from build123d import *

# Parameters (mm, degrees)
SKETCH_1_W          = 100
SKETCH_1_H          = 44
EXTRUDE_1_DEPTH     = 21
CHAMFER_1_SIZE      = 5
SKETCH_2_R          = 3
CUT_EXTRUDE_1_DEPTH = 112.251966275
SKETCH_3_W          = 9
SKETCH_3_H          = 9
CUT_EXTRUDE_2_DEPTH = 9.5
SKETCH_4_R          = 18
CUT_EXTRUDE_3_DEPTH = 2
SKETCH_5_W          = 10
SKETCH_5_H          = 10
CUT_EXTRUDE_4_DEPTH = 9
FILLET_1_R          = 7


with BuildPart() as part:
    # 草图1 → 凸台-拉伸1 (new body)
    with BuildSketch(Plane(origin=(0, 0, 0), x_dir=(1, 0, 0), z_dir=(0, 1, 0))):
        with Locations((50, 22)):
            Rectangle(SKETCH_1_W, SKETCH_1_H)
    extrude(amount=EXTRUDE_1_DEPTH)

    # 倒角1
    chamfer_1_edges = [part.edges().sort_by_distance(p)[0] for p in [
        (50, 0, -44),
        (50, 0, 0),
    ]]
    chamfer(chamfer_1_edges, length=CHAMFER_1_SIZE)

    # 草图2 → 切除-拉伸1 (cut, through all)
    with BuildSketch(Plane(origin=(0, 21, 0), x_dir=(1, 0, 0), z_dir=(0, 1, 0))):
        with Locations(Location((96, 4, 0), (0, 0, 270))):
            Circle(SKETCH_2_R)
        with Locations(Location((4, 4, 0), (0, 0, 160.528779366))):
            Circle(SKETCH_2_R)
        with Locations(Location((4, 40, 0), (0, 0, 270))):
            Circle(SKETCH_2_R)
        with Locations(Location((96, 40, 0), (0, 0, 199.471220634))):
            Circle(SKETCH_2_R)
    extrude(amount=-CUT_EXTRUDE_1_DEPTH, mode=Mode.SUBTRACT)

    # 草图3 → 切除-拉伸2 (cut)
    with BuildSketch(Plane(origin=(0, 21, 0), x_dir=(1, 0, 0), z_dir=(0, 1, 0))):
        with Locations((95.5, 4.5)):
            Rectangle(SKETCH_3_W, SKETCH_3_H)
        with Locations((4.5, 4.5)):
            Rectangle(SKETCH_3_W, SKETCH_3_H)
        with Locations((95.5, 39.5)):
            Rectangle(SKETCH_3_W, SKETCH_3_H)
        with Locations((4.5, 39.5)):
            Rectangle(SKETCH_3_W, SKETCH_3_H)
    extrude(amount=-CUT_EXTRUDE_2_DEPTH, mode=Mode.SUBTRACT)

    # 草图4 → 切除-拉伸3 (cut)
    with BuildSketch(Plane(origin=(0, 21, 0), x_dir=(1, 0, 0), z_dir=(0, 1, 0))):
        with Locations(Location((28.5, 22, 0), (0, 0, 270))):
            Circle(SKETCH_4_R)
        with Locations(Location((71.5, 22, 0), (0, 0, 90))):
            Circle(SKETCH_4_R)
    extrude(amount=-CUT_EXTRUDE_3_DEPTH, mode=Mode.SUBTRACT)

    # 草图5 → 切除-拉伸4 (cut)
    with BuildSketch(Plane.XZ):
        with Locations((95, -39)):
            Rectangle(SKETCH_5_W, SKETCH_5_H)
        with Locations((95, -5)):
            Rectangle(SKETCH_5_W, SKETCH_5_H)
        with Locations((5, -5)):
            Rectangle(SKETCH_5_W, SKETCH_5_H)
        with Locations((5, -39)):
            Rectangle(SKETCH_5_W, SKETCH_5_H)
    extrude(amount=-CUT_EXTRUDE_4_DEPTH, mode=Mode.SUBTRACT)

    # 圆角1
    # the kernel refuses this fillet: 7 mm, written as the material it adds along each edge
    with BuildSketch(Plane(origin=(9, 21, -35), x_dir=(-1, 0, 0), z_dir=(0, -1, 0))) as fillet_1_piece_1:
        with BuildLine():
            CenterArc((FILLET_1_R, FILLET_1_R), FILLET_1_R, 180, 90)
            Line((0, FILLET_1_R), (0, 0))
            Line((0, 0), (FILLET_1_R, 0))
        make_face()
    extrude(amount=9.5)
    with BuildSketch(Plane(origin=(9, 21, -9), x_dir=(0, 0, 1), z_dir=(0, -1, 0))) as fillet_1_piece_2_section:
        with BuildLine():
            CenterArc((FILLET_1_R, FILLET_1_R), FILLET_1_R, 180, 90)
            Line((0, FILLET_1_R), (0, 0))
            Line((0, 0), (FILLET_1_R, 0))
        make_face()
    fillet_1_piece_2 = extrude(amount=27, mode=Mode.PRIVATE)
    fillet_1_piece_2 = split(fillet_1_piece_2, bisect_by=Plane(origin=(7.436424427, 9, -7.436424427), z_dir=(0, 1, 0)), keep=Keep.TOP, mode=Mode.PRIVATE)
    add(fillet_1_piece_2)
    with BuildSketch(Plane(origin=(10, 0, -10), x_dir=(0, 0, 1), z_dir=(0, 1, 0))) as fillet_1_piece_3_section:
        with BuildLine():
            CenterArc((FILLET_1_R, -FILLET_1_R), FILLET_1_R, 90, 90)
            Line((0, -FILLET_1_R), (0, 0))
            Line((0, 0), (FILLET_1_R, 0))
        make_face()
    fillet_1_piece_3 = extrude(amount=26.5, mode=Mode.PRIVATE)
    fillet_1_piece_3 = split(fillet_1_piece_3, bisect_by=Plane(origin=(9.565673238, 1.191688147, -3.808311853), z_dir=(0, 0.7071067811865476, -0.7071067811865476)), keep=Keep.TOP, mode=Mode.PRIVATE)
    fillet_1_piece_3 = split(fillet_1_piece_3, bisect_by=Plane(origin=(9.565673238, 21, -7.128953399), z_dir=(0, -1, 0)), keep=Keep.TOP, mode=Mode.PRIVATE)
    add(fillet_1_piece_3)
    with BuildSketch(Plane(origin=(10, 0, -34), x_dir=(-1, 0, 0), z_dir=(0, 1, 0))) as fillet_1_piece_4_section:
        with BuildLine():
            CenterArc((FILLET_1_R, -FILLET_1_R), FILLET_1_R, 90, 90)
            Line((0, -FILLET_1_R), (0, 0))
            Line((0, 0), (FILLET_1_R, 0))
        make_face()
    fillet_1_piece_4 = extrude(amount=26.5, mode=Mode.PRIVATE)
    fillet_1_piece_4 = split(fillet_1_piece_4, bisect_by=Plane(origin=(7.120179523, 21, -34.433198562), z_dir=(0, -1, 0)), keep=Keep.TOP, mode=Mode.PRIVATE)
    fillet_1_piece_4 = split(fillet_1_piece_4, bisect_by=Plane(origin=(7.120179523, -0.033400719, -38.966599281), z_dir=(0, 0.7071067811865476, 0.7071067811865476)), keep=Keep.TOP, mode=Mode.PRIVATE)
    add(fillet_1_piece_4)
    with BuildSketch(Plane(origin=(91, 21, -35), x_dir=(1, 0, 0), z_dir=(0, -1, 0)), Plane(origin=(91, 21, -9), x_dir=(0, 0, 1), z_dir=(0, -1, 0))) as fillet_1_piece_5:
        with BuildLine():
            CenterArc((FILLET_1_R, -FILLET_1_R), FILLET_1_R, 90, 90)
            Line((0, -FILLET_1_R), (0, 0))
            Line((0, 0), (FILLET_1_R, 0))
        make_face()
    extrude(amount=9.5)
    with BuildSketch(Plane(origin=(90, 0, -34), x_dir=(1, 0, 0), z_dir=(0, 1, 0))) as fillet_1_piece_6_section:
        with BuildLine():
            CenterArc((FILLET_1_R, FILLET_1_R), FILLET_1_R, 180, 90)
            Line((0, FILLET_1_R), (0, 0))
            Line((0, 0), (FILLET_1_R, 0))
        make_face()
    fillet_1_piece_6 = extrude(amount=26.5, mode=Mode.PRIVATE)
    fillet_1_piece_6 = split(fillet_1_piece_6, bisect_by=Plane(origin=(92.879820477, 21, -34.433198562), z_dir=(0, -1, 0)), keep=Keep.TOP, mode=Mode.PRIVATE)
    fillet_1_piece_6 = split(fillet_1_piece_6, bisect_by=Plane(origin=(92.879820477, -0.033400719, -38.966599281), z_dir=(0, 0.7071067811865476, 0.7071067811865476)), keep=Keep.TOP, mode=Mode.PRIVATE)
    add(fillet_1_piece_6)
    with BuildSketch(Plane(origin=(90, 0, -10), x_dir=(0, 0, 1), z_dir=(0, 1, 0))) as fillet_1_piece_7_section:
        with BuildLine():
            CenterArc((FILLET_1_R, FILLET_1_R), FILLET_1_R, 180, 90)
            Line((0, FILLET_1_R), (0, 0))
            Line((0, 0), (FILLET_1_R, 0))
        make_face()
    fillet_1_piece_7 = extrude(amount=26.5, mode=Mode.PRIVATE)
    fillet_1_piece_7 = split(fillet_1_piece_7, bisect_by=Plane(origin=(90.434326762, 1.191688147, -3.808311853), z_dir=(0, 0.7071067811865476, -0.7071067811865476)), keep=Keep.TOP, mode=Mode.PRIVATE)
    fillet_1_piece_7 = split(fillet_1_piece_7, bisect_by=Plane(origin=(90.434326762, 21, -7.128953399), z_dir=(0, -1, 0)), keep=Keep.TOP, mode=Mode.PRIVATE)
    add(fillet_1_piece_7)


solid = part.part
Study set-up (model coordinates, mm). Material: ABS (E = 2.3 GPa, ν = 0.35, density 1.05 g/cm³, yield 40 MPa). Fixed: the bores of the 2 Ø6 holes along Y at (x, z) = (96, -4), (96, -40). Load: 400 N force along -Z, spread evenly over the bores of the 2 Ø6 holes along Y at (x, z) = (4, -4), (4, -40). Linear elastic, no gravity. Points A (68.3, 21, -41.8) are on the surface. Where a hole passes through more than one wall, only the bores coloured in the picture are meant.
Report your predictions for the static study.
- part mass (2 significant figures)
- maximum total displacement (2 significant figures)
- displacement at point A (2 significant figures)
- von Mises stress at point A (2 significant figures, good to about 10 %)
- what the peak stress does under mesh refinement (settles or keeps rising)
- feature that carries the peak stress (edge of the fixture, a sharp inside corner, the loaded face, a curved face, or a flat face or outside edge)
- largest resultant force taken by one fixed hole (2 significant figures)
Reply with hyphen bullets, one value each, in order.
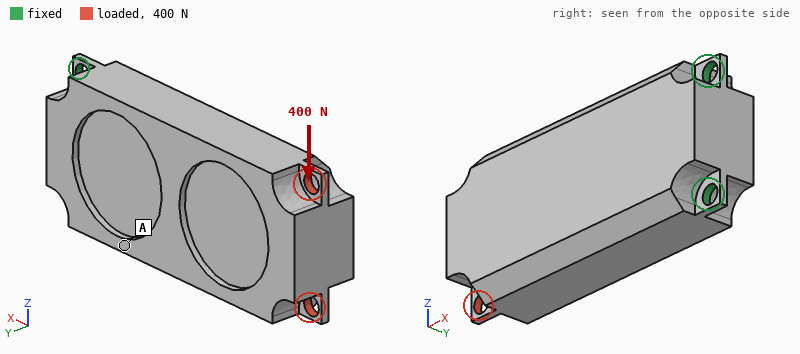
- 84 g
- 0.93 mm
- 0.21 mm
- 4.0 MPa
- keeps rising
- edge of the fixture
- 1.0 kN
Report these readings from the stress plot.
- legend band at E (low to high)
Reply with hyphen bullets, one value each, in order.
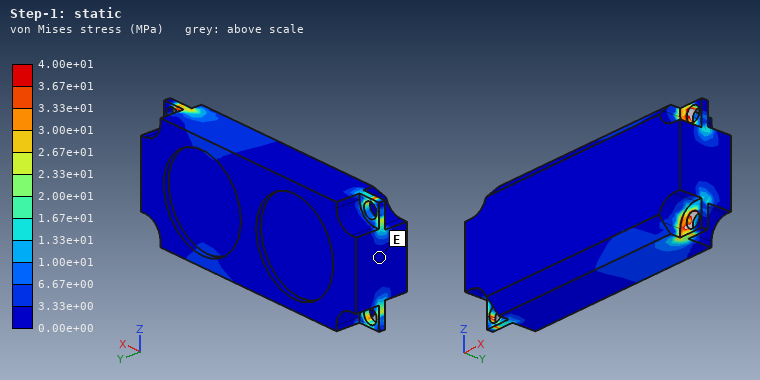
- 0.00e+00 to 3.33e+00 MPa
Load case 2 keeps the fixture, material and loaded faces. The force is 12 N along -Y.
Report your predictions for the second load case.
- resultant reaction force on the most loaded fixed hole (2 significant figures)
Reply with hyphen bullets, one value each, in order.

- 7.3 N
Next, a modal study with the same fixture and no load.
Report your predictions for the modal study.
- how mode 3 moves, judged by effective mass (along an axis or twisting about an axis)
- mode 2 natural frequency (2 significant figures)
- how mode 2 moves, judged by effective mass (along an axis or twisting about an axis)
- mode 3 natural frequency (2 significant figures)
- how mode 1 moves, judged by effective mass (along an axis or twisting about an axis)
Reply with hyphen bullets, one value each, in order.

- twisting about X
- 700 Hz
- along Z
- 1500 Hz
- along Y
